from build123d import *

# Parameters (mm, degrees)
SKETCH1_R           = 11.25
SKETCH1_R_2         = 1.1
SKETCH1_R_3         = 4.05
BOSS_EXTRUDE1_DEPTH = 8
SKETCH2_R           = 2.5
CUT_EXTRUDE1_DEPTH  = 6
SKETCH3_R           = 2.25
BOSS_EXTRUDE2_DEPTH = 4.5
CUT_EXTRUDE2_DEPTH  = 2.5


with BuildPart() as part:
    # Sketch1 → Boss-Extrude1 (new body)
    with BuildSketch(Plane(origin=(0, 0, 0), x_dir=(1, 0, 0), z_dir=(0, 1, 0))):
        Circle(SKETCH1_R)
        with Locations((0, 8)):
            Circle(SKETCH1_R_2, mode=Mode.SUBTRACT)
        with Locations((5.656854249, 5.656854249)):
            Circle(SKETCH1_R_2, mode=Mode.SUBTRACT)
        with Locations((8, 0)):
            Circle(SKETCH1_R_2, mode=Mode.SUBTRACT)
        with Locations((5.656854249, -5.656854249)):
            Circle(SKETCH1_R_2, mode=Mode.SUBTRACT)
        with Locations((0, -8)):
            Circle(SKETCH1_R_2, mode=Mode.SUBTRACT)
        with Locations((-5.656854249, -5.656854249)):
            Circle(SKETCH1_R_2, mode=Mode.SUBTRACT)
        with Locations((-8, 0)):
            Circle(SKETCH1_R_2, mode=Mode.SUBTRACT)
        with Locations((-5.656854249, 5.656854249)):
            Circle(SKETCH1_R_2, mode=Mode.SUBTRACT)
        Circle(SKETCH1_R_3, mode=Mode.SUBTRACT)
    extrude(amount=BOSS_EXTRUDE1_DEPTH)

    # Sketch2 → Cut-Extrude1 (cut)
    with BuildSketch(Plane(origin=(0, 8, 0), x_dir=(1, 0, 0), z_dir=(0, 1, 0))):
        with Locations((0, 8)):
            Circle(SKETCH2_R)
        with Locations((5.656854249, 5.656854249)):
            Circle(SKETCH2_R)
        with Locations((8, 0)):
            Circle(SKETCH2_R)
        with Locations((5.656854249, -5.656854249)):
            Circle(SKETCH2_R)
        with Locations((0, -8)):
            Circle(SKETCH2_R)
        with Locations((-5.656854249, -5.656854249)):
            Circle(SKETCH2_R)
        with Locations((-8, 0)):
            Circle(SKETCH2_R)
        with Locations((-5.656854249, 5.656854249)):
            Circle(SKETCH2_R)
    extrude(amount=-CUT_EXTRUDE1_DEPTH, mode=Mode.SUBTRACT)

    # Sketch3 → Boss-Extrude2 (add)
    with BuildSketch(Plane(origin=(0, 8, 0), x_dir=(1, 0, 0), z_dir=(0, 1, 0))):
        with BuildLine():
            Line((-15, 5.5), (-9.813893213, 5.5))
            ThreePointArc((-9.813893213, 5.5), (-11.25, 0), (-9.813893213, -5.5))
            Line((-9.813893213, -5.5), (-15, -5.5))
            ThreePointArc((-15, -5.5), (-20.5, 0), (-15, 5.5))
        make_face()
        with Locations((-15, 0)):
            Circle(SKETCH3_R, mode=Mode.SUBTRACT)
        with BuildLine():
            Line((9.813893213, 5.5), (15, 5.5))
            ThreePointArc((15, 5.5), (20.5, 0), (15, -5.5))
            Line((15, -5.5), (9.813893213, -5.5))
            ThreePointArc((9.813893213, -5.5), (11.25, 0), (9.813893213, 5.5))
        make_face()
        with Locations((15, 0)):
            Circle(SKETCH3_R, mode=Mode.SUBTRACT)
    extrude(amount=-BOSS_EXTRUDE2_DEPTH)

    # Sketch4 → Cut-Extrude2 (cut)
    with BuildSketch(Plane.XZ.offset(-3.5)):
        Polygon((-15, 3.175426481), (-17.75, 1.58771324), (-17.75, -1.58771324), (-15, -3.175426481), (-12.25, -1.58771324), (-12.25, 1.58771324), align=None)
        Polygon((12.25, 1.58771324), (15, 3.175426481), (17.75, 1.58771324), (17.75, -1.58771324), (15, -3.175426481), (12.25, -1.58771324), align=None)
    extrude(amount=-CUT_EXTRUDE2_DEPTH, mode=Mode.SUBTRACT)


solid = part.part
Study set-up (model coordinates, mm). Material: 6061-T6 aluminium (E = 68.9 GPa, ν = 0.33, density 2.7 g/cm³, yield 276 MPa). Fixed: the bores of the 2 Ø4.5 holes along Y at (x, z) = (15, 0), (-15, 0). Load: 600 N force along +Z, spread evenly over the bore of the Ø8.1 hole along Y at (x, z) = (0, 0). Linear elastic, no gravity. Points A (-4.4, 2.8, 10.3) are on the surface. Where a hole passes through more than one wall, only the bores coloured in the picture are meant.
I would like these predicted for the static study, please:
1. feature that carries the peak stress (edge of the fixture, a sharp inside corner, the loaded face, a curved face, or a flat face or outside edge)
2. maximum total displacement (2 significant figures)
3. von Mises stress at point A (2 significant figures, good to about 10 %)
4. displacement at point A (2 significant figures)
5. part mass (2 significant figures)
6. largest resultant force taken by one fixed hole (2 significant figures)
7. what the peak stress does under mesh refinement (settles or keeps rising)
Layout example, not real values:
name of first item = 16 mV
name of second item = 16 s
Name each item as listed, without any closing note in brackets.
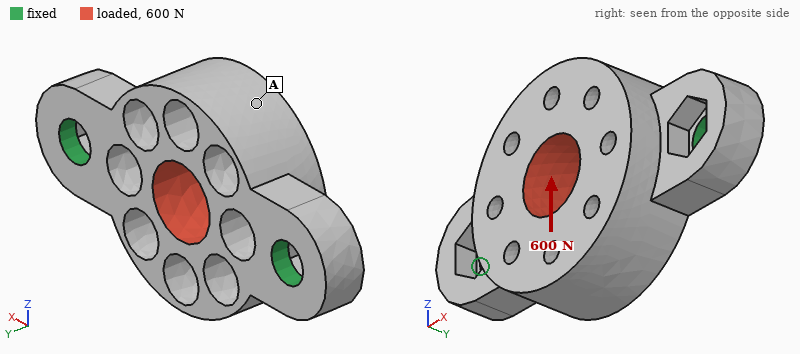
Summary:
feature that carries the peak stress = edge of the fixture
maximum total displacement = 16 µm
von Mises stress at point A = 12 MPa
displacement at point A = 13 µm
part mass = 6.5 g
largest resultant force taken by one fixed hole = 300 N
what the peak stress does under mesh refinement = keeps rising
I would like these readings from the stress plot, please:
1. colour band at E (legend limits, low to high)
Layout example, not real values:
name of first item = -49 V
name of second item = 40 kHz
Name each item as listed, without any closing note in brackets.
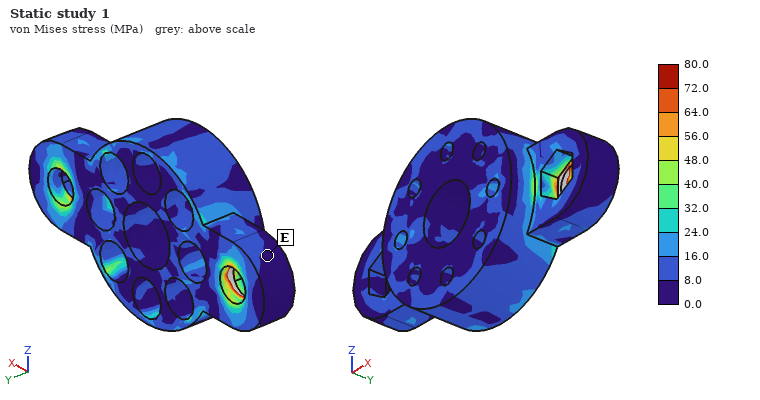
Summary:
colour band at E = 0.0 to 8.0 MPa
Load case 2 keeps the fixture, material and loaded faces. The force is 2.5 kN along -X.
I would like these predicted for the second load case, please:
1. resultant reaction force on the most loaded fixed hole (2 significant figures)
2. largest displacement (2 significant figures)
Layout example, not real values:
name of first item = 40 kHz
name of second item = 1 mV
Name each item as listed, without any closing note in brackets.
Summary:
resultant reaction force on the most loaded fixed hole = 1.3 kN
largest displacement = 14 µm
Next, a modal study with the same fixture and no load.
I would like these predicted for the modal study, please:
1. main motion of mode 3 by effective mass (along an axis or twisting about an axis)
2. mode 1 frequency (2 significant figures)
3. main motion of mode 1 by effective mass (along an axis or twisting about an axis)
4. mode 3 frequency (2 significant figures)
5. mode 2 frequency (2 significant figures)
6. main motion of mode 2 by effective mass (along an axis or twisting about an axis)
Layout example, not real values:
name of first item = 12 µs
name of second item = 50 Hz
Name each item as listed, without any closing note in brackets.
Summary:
main motion of mode 3 by effective mass = along Z
mode 1 frequency = 12 kHz
main motion of mode 1 by effective mass = along Z
mode 3 frequency = 29 kHz
mode 2 frequency = 20 kHz
main motion of mode 2 by effective mass = along Y
